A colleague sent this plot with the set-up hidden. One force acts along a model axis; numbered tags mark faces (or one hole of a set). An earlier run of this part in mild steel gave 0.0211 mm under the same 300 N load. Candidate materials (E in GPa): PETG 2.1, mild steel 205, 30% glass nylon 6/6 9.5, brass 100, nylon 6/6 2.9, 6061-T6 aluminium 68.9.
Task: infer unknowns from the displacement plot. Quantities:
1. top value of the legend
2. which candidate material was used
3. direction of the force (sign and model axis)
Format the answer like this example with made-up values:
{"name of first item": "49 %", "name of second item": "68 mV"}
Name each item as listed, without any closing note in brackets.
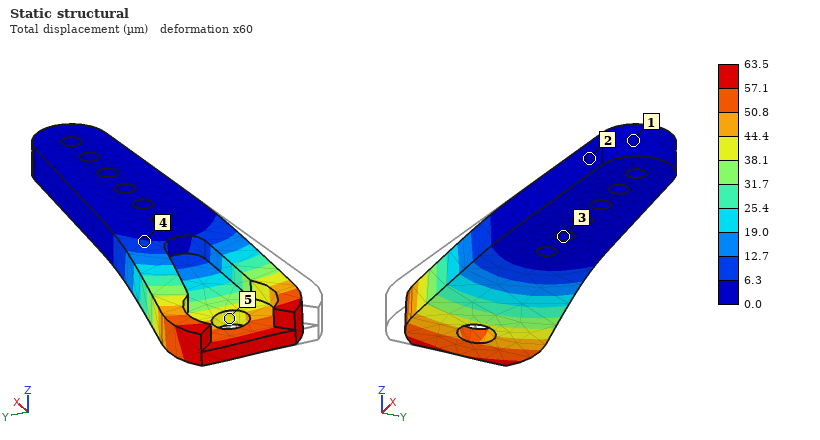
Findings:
{"top value of the legend": "63.5 µm", "which candidate material was used": "6061-T6 aluminium", "direction of the force": "+Y"}
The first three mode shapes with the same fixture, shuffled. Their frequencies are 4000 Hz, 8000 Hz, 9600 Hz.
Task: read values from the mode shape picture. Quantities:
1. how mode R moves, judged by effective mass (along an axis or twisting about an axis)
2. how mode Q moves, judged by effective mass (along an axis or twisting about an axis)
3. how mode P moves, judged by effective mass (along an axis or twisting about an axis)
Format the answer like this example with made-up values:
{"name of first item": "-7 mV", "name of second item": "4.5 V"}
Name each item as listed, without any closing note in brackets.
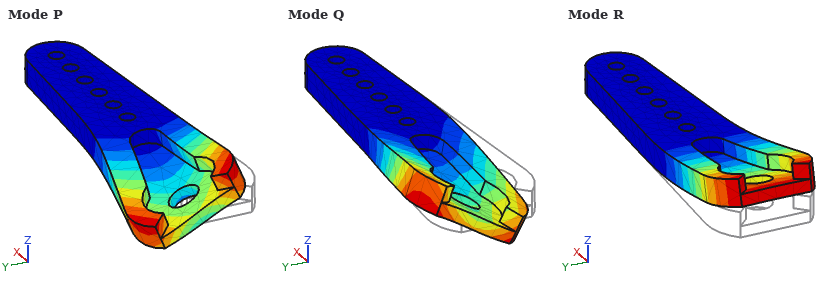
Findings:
{"how mode R moves, judged by effective mass": "along Z", "how mode Q moves, judged by effective mass": "along Y", "how mode P moves, judged by effective mass": "along Y"}
